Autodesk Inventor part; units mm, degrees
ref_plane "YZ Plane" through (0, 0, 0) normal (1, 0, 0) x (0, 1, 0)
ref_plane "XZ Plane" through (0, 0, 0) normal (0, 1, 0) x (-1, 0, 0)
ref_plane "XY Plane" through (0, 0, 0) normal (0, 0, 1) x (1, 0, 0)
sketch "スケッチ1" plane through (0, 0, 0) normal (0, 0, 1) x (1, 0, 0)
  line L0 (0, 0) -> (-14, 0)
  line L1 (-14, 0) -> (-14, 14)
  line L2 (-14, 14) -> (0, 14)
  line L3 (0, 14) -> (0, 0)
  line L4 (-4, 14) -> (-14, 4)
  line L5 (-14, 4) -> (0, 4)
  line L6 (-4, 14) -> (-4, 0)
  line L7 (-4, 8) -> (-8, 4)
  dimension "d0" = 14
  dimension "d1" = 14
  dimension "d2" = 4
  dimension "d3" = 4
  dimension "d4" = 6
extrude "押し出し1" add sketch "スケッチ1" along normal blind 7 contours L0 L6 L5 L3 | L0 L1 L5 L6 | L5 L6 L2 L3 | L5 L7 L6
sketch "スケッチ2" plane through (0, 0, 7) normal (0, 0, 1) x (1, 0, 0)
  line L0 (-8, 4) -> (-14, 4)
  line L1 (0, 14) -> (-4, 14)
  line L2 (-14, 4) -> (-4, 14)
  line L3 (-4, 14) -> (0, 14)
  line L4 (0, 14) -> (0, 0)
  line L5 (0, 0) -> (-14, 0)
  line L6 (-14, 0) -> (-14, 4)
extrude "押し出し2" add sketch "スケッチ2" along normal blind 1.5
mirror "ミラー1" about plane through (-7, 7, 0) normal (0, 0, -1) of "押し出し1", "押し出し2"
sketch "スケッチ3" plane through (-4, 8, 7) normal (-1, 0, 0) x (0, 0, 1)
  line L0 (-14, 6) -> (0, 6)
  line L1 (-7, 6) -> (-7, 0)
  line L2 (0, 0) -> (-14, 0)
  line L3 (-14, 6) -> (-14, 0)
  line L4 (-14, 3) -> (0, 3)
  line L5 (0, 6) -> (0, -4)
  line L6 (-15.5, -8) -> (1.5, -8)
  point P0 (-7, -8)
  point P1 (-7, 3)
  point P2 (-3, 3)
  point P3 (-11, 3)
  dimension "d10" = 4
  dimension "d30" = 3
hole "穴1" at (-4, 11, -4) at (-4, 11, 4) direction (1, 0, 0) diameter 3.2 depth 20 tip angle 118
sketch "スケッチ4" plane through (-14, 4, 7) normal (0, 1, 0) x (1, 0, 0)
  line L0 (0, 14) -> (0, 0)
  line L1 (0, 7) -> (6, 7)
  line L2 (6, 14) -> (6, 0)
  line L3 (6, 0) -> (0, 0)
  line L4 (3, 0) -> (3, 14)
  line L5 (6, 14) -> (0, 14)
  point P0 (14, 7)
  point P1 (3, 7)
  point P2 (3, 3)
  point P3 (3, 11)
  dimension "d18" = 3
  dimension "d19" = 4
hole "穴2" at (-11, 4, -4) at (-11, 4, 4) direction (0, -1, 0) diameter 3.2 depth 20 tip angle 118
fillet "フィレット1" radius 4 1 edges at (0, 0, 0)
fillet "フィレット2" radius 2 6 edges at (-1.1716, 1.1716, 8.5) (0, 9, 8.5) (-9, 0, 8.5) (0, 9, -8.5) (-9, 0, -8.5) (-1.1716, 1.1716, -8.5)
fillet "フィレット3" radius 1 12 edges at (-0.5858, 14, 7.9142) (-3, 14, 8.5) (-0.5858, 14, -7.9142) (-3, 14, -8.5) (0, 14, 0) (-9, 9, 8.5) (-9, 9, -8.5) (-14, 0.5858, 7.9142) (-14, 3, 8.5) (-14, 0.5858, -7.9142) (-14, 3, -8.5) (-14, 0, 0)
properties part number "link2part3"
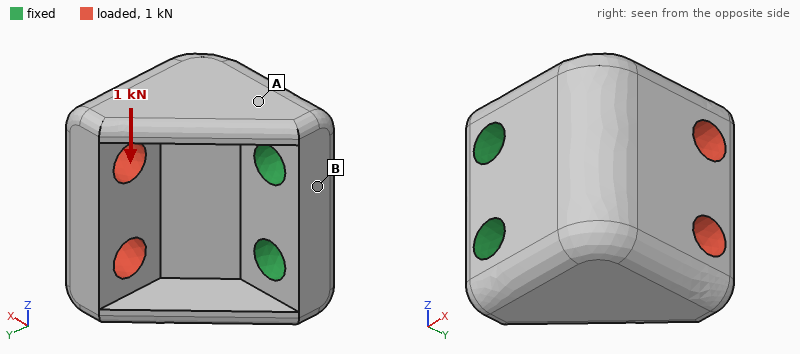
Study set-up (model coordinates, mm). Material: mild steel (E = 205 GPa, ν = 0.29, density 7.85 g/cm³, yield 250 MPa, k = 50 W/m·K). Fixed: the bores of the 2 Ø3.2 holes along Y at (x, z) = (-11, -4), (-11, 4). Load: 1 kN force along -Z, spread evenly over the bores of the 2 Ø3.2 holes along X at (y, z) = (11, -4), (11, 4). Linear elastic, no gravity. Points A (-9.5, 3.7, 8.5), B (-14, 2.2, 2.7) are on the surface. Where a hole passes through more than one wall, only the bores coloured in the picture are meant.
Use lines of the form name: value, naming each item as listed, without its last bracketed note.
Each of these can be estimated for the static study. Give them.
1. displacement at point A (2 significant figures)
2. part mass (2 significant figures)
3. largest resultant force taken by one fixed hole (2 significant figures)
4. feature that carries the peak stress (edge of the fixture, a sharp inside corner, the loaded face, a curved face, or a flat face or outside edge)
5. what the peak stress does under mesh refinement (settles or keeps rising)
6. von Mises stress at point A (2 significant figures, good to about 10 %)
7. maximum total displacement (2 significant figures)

displacement at point A: 2.2 µm
part mass: 13 g
largest resultant force taken by one fixed hole: 1.2 kN
feature that carries the peak stress: edge of the fixture
what the peak stress does under mesh refinement: keeps rising
von Mises stress at point A: 59 MPa
maximum total displacement: 14 µm
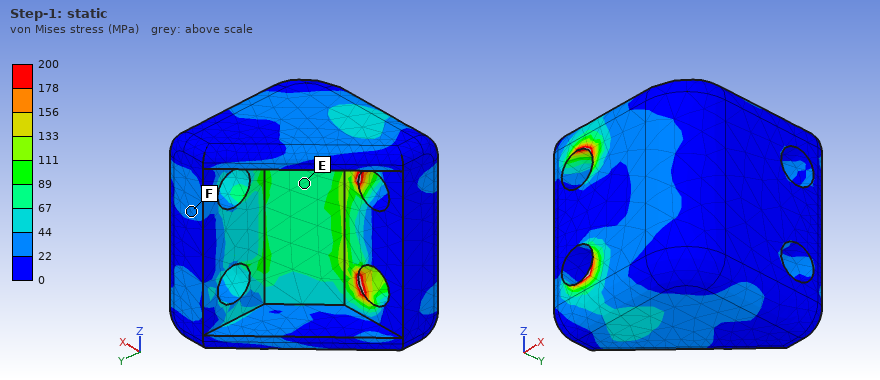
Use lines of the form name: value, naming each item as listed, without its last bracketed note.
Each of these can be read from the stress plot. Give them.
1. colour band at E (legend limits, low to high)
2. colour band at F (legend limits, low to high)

colour band at E: 67 to 89 MPa
colour band at F: 22 to 44 MPa
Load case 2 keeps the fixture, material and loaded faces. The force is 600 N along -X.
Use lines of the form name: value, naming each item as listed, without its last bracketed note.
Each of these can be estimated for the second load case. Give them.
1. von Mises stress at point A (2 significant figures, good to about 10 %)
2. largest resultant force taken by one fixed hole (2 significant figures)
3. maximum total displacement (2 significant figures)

von Mises stress at point A: 19 MPa
largest resultant force taken by one fixed hole: 300 N
maximum total displacement: 16 µm
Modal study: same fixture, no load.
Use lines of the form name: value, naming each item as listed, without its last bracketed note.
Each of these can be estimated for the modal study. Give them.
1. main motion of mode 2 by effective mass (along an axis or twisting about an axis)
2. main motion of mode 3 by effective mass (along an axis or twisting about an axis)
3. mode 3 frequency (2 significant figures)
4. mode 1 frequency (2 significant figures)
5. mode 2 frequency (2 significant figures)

main motion of mode 2 by effective mass: along Z
main motion of mode 3 by effective mass: along Z
mode 3 frequency: 36 kHz
mode 1 frequency: 15 kHz
mode 2 frequency: 23 kHz
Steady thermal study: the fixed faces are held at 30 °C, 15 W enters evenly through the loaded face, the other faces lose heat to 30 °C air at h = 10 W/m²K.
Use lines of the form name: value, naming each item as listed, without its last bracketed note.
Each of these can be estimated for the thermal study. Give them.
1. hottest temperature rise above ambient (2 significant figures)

hottest temperature rise above ambient: 57 K
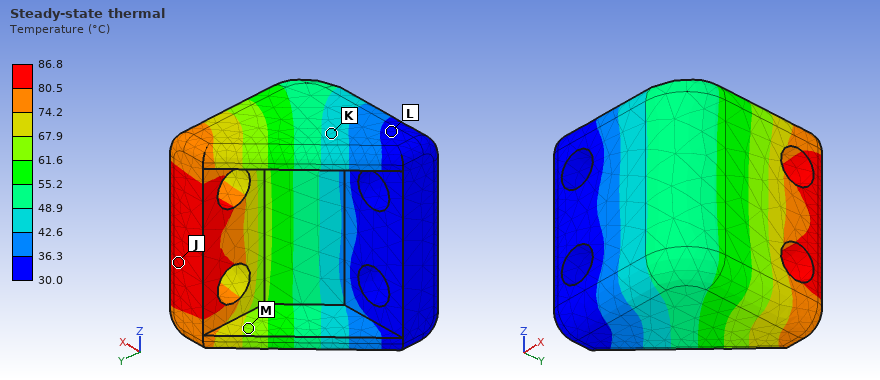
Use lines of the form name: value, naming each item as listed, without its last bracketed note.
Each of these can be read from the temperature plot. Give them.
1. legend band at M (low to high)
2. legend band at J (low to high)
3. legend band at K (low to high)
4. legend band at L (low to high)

legend band at M: 61.6 to 67.9 °C
legend band at J: 80.5 to 86.8 °C
legend band at K: 42.6 to 48.9 °C
legend band at L: 30.0 to 36.3 °C
